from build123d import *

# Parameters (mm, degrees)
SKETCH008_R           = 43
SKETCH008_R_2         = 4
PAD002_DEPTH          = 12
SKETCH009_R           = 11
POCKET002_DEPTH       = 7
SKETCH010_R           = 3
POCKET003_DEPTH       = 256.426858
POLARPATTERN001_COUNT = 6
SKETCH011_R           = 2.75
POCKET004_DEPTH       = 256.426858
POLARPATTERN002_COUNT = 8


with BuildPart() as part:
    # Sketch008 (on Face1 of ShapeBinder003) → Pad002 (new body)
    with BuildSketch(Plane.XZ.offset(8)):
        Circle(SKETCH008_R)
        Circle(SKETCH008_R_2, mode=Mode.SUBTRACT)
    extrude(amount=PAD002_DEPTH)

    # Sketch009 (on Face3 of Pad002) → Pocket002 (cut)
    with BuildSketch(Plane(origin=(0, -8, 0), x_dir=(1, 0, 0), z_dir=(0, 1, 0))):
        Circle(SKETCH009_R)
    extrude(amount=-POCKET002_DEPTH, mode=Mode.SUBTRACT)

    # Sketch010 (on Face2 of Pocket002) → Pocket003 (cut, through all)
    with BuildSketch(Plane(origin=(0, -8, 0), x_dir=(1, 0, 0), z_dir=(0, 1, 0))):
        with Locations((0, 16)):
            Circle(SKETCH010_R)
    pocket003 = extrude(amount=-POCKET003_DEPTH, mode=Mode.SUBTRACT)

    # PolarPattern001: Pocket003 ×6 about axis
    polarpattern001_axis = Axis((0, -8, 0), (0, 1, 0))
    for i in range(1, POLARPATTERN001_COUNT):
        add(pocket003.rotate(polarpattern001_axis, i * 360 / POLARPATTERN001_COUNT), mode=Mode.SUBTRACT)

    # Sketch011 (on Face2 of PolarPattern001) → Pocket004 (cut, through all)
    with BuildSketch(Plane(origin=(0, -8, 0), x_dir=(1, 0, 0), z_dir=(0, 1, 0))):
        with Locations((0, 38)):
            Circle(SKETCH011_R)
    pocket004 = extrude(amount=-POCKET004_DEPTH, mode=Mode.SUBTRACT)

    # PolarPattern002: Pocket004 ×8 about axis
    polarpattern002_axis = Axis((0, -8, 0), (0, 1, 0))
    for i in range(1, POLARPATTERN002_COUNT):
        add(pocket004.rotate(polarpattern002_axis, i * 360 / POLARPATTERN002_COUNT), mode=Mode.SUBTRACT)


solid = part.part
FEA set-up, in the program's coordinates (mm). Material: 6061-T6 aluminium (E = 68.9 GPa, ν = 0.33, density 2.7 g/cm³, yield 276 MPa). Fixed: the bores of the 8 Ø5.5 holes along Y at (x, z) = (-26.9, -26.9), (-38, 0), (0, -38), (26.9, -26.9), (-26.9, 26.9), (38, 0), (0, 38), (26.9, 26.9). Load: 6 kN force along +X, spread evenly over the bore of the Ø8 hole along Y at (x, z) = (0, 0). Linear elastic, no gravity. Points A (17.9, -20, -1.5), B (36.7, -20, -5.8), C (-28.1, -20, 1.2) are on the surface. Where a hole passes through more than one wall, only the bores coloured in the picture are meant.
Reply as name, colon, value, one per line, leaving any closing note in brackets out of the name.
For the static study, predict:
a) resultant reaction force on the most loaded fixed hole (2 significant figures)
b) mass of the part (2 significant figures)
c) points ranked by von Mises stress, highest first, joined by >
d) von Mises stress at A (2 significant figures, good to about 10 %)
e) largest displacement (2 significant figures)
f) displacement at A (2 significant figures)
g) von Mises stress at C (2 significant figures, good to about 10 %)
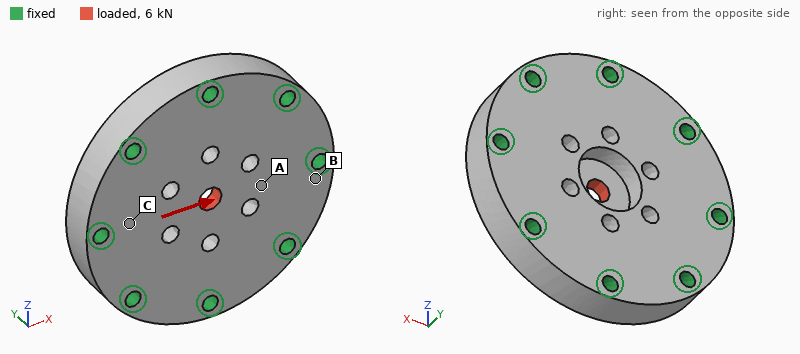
resultant reaction force on the most loaded fixed hole: 1.3 kN
mass of the part: 170 g
points ranked by von Mises stress, highest first, joined by >: A > C > B
von Mises stress at A: 18 MPa
largest displacement: 9.6 µm
displacement at A: 3.2 µm
von Mises stress at C: 11 MPa
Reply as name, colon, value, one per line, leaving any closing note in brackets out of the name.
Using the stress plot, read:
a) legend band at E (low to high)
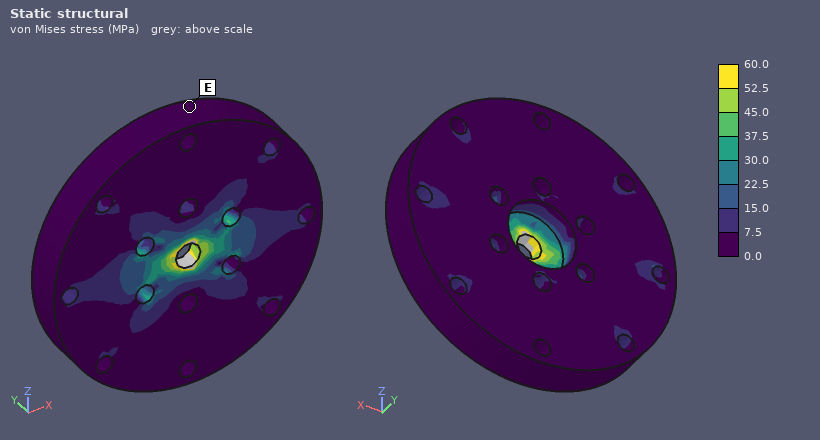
legend band at E: 0.0 to 7.5 MPa
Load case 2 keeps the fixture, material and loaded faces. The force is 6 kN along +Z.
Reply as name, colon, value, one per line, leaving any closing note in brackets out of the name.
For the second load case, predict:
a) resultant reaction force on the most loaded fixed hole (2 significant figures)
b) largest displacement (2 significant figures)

resultant reaction force on the most loaded fixed hole: 1.3 kN
largest displacement: 9.7 µm
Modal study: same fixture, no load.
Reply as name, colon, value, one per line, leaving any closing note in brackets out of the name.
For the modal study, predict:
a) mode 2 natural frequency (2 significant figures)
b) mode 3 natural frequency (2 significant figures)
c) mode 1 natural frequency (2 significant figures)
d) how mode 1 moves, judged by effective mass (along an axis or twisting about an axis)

mode 2 natural frequency: 25 kHz
mode 3 natural frequency: 25 kHz
mode 1 natural frequency: 16 kHz
how mode 1 moves, judged by effective mass: along Y
